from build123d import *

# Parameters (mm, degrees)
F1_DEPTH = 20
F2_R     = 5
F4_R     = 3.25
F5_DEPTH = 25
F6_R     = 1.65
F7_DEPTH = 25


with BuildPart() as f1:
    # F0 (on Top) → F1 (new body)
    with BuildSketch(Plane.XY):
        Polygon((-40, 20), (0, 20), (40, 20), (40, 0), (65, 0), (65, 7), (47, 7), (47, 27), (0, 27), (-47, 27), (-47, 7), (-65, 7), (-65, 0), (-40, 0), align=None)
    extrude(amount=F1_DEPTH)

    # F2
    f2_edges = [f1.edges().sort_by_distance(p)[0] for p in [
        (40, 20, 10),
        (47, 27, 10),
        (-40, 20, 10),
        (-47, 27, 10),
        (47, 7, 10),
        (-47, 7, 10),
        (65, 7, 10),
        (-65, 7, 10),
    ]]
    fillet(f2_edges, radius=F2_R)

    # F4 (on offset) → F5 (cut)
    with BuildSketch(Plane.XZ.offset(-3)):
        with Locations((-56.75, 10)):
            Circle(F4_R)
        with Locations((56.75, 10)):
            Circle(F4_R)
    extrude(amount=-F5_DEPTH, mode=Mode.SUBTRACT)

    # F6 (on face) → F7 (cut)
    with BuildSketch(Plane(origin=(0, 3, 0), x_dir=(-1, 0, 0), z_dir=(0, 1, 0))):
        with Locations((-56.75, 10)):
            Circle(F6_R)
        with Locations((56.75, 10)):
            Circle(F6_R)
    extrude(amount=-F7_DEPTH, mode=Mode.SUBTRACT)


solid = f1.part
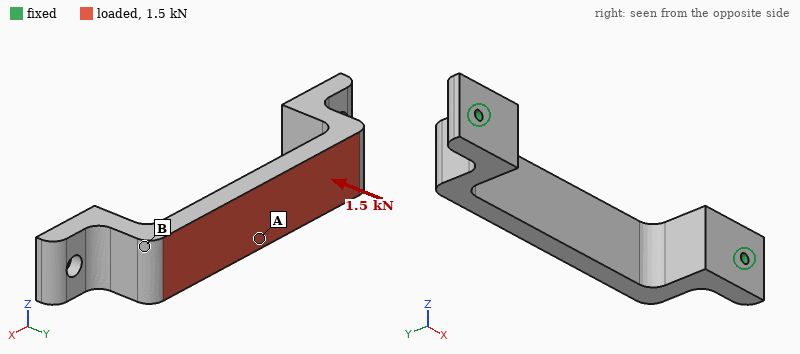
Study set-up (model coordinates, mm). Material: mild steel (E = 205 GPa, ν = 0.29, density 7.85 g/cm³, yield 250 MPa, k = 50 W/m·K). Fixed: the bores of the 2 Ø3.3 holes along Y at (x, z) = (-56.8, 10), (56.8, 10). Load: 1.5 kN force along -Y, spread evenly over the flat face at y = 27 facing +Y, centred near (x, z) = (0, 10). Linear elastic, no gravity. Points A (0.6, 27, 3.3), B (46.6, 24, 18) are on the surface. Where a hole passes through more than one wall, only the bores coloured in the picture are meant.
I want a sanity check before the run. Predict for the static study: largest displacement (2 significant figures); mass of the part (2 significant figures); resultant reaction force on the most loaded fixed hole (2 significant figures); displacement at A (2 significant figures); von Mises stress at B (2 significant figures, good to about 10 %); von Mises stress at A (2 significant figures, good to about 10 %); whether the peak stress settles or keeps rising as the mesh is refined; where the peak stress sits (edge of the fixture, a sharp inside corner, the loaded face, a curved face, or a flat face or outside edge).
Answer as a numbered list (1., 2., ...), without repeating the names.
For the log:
1. 27 µm
2. 180 g
3. 1.2 kN
4. 27 µm
5. 7.8 MPa
6. 40 MPa
7. keeps rising
8. edge of the fixture
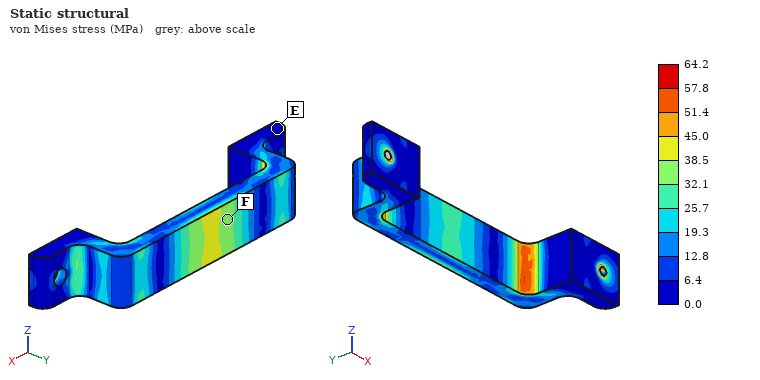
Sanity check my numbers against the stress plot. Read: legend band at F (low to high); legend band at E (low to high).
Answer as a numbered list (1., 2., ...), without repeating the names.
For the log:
1. 32.1 to 38.5 MPa
2. 0.0 to 6.4 MPa
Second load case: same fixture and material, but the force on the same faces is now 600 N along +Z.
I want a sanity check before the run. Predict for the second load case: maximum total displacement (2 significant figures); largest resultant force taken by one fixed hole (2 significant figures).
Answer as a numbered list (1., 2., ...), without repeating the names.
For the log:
1. 60 µm
2. 300 N
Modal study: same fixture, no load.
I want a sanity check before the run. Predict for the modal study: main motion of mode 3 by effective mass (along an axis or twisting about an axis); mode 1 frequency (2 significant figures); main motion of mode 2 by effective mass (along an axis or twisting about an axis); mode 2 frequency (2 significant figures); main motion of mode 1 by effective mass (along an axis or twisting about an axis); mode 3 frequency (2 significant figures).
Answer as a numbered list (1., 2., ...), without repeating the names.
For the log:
1. twisting about Y
2. 1700 Hz
3. along X
4. 3200 Hz
5. along Z
6. 4300 Hz
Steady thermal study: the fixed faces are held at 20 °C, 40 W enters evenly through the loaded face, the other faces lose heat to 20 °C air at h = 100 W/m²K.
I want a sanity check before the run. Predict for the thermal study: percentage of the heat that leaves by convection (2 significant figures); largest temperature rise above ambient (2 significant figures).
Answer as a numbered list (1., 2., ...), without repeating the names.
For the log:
1. 65 %
2. 72 K
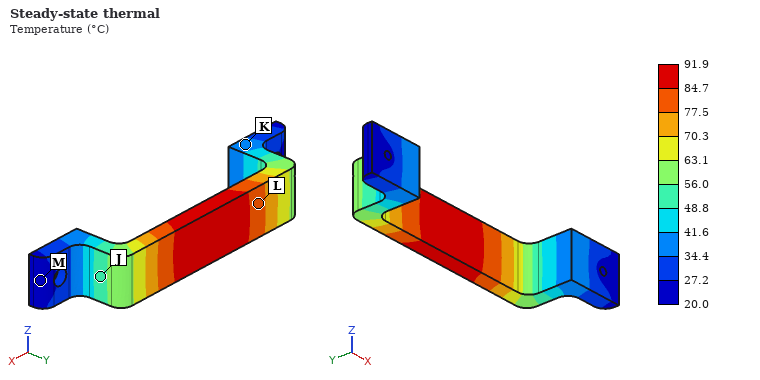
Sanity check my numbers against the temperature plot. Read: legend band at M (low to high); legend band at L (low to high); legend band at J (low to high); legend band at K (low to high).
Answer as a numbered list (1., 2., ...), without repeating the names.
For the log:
1. 20.0 to 27.2 °C
2. 77.5 to 84.7 °C
3. 48.8 to 56.0 °C
4. 34.4 to 41.6 °C
